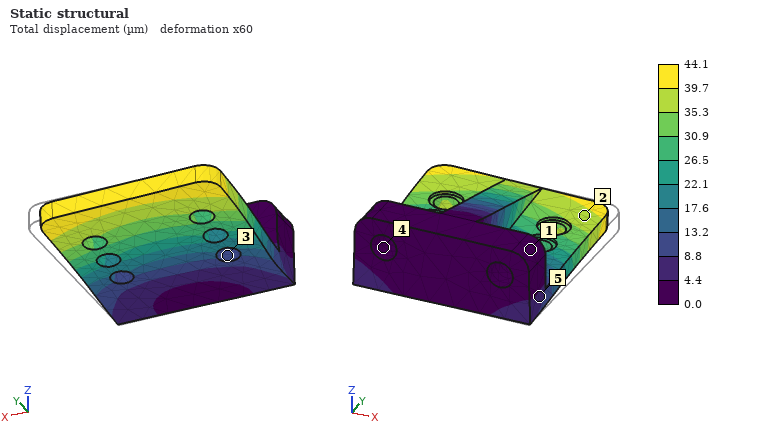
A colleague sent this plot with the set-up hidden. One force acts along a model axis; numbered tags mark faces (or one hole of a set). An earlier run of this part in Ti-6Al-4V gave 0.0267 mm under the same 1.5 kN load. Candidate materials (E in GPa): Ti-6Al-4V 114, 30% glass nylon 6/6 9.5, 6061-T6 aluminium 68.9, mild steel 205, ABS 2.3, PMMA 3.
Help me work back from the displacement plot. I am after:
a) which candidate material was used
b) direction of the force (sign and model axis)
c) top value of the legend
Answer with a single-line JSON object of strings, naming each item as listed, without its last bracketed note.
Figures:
{"which candidate material was used": "6061-T6 aluminium", "direction of the force": "-X", "top value of the legend": "44.1 µm"}
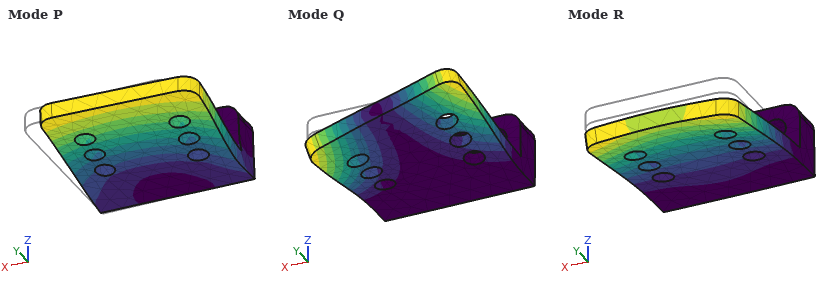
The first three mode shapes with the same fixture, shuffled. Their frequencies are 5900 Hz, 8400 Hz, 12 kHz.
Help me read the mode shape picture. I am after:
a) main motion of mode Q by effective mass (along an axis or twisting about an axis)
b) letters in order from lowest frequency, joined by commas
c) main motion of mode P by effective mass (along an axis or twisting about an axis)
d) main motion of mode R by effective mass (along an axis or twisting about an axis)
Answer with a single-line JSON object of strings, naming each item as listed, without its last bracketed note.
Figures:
{"main motion of mode Q by effective mass": "twisting about Y", "letters in order from lowest frequency, joined by commas": "R, Q, P", "main motion of mode P by effective mass": "along X", "main motion of mode R by effective mass": "along Z"}
